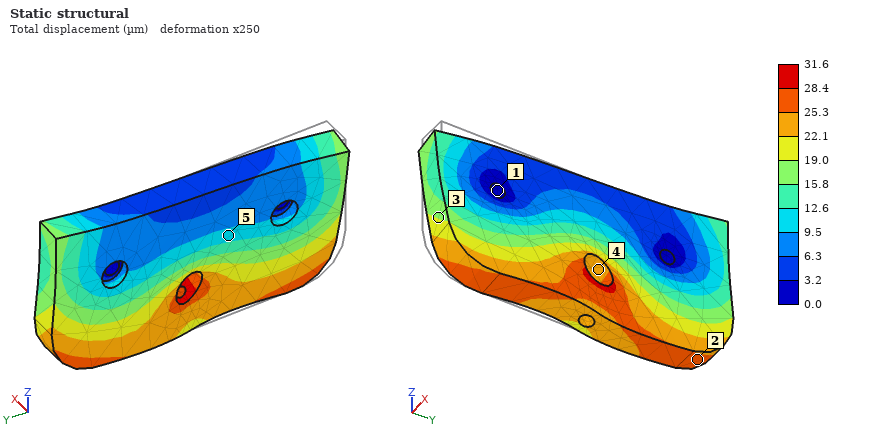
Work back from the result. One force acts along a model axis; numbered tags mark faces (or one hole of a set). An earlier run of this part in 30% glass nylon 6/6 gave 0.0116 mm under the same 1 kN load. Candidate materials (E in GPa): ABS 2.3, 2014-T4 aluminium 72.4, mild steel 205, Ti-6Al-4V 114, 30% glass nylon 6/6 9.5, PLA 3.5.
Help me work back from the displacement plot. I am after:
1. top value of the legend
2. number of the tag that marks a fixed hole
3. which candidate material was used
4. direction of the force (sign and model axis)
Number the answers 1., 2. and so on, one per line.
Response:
1. 31.6 µm
2. 1
3. PLA
4. +Y
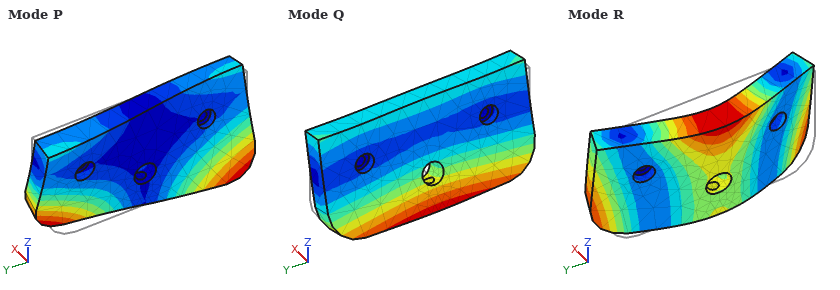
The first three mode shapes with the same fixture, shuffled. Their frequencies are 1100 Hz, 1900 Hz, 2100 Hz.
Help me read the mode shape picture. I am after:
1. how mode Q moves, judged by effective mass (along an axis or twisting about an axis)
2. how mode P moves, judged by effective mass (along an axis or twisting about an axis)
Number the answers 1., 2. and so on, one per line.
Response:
1. along X
2. twisting about Z
